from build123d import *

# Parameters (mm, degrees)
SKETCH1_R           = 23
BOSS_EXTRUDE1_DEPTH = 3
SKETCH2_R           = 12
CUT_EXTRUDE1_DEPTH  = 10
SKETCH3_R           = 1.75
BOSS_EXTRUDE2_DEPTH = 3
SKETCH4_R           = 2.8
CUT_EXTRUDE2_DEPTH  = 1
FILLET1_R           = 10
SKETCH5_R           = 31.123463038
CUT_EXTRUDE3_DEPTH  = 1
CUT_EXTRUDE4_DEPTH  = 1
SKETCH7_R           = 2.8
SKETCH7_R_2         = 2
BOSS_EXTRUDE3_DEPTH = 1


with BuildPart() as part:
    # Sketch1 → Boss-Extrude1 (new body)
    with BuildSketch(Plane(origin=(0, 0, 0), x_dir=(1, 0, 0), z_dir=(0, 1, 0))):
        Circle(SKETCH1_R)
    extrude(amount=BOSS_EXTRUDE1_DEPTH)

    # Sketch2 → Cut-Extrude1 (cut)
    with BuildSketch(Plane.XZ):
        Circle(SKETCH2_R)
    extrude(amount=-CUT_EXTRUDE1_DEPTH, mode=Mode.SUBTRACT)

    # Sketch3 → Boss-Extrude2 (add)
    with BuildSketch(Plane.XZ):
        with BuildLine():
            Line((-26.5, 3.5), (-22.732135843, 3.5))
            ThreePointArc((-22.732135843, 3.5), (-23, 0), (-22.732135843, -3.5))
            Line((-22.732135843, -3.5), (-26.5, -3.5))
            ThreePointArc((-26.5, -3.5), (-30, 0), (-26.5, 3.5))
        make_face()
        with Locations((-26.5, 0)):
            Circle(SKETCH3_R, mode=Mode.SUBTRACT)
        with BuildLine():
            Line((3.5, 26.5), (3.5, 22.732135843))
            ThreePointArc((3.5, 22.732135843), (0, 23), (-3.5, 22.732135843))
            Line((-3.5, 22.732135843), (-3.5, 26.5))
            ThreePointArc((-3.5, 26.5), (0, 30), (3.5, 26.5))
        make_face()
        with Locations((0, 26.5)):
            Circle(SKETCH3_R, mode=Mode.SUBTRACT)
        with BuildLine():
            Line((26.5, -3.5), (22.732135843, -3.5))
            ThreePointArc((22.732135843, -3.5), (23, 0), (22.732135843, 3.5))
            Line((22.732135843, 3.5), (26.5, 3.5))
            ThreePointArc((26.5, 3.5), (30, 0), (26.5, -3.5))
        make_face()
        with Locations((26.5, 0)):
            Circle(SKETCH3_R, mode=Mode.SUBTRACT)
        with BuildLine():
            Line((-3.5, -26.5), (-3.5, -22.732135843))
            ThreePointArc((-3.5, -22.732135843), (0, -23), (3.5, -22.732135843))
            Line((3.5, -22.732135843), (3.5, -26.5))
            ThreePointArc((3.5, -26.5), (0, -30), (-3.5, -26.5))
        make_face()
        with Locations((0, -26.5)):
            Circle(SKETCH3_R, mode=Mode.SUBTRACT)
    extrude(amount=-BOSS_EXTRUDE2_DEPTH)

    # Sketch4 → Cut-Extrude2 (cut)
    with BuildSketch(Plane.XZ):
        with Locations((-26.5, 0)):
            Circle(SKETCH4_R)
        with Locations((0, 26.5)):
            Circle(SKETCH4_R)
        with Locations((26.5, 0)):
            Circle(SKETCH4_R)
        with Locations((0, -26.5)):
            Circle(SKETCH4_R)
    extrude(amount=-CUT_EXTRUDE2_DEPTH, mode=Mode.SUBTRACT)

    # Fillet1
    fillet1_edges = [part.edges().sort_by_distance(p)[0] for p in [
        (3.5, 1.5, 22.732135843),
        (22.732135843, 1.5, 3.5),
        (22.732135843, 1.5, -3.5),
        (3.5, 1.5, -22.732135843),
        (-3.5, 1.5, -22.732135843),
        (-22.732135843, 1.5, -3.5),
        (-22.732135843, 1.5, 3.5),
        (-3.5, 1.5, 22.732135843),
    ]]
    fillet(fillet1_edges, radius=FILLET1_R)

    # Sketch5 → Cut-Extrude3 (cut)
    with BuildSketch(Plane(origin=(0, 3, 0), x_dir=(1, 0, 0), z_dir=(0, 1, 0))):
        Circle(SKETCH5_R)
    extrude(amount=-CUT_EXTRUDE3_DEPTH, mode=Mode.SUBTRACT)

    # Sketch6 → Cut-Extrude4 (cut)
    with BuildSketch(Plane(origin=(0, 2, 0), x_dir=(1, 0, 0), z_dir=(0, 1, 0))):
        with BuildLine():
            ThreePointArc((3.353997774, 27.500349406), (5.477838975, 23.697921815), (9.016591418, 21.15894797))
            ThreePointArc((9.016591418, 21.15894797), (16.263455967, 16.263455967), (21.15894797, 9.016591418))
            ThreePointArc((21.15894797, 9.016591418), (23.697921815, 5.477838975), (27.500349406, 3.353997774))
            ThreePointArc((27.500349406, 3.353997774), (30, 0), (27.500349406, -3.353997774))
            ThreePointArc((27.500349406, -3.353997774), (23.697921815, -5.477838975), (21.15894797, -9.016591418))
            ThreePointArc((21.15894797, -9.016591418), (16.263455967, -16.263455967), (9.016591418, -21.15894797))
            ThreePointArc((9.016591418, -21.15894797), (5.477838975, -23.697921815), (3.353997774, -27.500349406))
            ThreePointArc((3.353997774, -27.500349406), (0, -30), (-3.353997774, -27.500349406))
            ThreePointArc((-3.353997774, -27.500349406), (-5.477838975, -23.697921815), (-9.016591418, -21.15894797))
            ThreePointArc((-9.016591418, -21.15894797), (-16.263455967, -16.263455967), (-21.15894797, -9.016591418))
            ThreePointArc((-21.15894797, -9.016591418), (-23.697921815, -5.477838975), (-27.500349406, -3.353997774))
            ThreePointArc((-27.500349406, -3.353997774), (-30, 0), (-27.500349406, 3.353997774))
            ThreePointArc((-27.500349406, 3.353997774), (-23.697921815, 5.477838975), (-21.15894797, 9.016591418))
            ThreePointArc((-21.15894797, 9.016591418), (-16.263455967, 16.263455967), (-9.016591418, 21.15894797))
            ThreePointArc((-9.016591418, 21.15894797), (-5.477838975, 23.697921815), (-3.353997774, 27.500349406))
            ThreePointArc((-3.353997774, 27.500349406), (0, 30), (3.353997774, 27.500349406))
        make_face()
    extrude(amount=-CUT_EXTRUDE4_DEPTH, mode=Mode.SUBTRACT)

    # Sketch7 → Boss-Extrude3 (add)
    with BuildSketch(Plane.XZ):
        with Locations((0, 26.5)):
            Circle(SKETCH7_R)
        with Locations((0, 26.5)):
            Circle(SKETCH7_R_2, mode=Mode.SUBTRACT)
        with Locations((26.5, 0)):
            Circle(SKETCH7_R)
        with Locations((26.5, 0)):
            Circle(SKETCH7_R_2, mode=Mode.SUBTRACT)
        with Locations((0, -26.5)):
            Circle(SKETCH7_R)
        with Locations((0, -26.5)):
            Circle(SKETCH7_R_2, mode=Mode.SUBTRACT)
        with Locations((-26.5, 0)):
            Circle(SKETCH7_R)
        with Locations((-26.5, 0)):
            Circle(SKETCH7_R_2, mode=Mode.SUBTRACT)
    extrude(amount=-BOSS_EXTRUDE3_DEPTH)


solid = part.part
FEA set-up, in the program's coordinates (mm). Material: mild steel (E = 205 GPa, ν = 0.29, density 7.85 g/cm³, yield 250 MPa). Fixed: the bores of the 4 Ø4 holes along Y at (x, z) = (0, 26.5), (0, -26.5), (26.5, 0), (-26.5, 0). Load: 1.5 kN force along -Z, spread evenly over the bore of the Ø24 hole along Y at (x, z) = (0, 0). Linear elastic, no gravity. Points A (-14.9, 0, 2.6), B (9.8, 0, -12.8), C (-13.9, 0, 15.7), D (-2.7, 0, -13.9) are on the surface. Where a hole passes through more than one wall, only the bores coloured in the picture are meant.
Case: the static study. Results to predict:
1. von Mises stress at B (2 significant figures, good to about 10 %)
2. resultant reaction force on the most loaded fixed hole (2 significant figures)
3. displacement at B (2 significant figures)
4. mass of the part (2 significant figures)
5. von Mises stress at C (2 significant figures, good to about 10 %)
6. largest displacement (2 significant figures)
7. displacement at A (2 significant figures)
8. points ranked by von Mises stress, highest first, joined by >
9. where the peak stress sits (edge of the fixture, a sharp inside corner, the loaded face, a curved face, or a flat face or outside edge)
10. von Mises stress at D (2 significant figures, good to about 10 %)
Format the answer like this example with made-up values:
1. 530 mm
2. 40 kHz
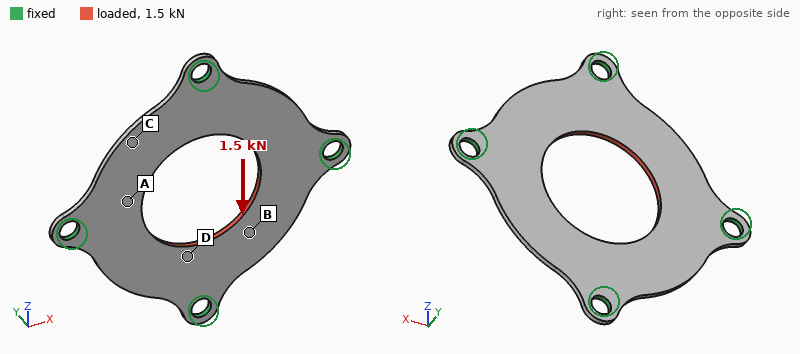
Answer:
1. 31 MPa
2. 510 N
3. 4.1 µm
4. 11 g
5. 17 MPa
6. 5.3 µm
7. 4.2 µm
8. D > B > C > A
9. edge of the fixture
10. 42 MPa
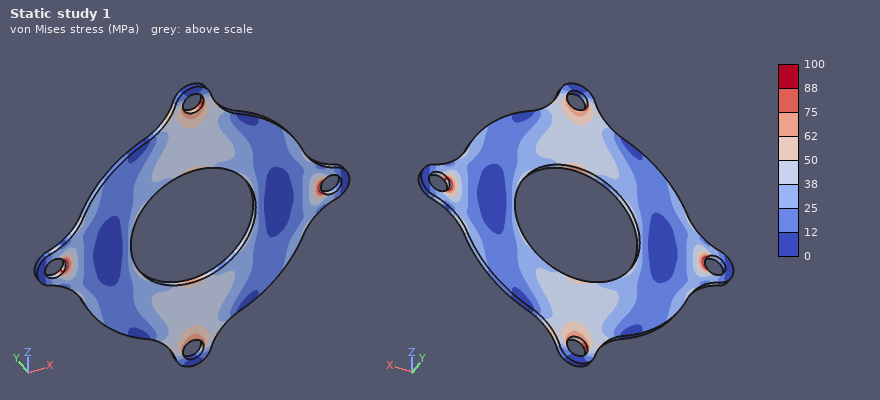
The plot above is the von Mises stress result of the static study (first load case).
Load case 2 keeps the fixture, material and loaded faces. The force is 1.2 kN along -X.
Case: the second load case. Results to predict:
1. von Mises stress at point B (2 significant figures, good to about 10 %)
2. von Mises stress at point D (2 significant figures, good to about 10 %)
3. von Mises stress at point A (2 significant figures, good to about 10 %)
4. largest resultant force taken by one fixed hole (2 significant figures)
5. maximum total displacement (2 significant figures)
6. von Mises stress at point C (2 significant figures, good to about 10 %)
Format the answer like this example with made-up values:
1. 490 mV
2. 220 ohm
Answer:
1. 16 MPa
2. 9.2 MPa
3. 33 MPa
4. 410 N
5. 4.2 µm
6. 16 MPa
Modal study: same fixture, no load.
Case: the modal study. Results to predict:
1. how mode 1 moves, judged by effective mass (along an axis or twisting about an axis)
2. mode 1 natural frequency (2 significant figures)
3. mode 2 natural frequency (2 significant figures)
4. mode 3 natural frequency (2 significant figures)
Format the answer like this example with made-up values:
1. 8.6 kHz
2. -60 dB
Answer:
1. along Y
2. 3600 Hz
3. 4400 Hz
4. 4400 Hz
